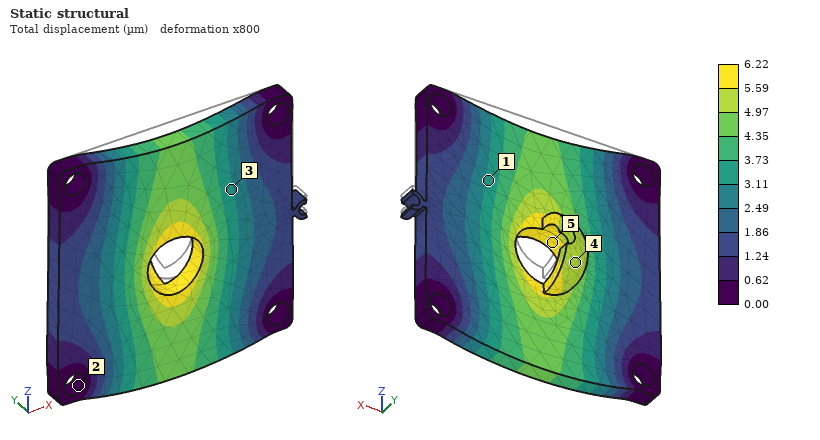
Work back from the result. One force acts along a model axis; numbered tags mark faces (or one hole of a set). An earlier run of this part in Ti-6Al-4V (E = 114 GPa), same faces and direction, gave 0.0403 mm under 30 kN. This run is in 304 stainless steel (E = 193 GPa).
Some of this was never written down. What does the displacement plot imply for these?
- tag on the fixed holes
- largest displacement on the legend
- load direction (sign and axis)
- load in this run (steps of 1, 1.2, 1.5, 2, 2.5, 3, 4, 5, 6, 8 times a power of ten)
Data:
2
6.22 µm
-Z
8 kN
